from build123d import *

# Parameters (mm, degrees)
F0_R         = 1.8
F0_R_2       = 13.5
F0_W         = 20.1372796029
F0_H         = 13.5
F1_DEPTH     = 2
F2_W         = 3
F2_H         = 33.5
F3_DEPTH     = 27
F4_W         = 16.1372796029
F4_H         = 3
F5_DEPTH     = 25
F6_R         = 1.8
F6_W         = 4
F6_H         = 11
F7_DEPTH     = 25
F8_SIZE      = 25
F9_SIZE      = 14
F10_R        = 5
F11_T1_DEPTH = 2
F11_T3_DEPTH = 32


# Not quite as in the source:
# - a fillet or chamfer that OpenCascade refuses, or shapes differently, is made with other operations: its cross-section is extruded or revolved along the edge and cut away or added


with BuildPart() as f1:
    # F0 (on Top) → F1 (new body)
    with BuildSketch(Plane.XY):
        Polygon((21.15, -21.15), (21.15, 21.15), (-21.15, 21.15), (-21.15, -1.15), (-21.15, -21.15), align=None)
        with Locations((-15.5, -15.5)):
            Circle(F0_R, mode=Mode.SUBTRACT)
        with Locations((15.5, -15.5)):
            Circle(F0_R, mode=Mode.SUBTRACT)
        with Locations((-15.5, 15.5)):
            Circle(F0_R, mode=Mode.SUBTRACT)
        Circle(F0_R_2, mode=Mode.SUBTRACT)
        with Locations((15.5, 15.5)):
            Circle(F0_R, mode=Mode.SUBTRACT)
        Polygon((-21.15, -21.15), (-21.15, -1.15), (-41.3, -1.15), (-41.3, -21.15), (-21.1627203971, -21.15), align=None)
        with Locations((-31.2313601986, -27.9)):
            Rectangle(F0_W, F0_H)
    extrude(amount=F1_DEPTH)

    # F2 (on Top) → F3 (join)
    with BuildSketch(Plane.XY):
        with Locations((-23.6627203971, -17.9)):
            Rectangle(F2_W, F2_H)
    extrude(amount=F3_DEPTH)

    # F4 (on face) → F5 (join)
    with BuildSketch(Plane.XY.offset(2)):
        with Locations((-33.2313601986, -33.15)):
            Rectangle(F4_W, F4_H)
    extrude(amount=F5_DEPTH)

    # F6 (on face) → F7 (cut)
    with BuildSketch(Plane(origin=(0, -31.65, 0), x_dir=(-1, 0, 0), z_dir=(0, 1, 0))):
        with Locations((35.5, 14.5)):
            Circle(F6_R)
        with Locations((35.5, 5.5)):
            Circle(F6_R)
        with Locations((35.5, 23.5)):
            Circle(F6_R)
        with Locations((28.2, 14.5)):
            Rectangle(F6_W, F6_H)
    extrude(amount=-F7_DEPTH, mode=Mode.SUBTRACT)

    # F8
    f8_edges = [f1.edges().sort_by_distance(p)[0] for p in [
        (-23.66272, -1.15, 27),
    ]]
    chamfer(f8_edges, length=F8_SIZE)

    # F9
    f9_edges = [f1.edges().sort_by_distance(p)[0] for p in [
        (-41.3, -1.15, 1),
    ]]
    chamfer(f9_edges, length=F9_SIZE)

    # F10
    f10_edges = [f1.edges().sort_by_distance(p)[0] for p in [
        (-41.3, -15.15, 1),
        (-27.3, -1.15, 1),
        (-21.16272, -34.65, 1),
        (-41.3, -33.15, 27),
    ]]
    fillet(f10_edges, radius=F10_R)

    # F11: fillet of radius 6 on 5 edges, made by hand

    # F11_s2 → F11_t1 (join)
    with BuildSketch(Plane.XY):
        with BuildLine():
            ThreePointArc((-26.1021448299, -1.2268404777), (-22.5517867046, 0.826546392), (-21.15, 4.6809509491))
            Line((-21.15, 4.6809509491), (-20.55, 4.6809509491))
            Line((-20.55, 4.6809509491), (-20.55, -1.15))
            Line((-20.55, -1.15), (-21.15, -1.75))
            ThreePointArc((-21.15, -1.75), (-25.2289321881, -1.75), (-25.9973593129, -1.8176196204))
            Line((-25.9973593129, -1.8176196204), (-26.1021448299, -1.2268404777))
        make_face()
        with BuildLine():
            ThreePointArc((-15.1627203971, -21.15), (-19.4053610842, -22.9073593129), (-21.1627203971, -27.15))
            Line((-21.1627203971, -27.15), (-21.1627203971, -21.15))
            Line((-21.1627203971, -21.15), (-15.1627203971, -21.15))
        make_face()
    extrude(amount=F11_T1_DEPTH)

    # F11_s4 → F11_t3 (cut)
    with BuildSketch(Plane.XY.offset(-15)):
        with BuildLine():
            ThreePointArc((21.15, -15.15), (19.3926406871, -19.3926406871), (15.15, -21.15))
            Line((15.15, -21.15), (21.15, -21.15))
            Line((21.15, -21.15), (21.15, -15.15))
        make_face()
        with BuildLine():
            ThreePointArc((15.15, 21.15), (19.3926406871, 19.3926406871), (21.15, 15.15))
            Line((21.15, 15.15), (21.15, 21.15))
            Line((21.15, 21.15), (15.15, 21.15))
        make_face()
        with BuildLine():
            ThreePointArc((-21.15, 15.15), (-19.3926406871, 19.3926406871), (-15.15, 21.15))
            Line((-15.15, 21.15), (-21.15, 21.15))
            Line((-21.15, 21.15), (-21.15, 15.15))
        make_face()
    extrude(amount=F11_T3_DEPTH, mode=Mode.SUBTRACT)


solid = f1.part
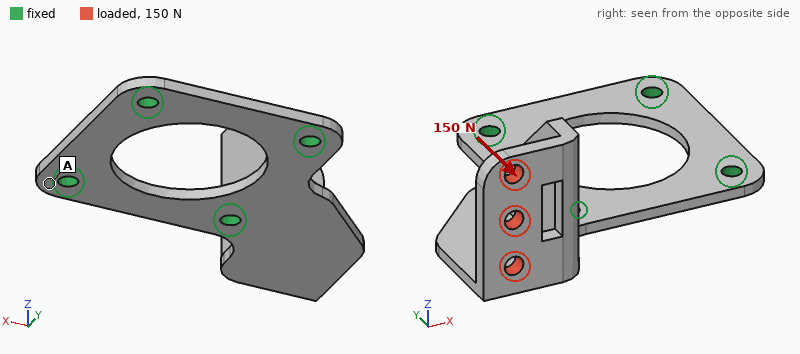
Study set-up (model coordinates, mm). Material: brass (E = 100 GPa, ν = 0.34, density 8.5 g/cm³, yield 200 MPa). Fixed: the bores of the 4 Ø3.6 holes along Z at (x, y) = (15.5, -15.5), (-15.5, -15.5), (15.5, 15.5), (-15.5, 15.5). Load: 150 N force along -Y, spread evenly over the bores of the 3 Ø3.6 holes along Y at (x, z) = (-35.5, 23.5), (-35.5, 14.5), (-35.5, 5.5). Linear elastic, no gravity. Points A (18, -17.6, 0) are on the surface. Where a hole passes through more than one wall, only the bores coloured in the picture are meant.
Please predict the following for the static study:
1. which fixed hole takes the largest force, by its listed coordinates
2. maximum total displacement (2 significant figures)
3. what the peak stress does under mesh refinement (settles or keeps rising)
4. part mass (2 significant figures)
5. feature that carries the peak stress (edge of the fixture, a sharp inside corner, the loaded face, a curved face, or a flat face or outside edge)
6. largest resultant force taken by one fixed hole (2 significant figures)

(-15.5, 15.5)
0.13 mm
keeps rising
51 g
edge of the fixture
150 N
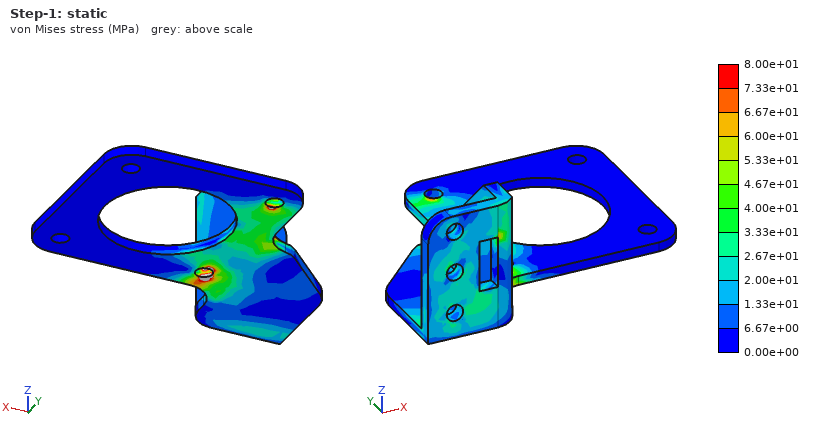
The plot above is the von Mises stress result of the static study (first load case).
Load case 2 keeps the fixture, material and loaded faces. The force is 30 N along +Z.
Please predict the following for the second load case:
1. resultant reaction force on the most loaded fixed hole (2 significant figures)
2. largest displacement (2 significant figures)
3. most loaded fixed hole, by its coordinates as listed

43 N
0.11 mm
(-15.5, -15.5)
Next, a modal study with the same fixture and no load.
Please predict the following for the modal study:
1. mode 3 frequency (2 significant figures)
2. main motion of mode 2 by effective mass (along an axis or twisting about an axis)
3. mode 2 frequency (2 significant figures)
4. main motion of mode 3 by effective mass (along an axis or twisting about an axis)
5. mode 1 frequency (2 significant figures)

4100 Hz
along Y
1500 Hz
along Z
720 Hz
